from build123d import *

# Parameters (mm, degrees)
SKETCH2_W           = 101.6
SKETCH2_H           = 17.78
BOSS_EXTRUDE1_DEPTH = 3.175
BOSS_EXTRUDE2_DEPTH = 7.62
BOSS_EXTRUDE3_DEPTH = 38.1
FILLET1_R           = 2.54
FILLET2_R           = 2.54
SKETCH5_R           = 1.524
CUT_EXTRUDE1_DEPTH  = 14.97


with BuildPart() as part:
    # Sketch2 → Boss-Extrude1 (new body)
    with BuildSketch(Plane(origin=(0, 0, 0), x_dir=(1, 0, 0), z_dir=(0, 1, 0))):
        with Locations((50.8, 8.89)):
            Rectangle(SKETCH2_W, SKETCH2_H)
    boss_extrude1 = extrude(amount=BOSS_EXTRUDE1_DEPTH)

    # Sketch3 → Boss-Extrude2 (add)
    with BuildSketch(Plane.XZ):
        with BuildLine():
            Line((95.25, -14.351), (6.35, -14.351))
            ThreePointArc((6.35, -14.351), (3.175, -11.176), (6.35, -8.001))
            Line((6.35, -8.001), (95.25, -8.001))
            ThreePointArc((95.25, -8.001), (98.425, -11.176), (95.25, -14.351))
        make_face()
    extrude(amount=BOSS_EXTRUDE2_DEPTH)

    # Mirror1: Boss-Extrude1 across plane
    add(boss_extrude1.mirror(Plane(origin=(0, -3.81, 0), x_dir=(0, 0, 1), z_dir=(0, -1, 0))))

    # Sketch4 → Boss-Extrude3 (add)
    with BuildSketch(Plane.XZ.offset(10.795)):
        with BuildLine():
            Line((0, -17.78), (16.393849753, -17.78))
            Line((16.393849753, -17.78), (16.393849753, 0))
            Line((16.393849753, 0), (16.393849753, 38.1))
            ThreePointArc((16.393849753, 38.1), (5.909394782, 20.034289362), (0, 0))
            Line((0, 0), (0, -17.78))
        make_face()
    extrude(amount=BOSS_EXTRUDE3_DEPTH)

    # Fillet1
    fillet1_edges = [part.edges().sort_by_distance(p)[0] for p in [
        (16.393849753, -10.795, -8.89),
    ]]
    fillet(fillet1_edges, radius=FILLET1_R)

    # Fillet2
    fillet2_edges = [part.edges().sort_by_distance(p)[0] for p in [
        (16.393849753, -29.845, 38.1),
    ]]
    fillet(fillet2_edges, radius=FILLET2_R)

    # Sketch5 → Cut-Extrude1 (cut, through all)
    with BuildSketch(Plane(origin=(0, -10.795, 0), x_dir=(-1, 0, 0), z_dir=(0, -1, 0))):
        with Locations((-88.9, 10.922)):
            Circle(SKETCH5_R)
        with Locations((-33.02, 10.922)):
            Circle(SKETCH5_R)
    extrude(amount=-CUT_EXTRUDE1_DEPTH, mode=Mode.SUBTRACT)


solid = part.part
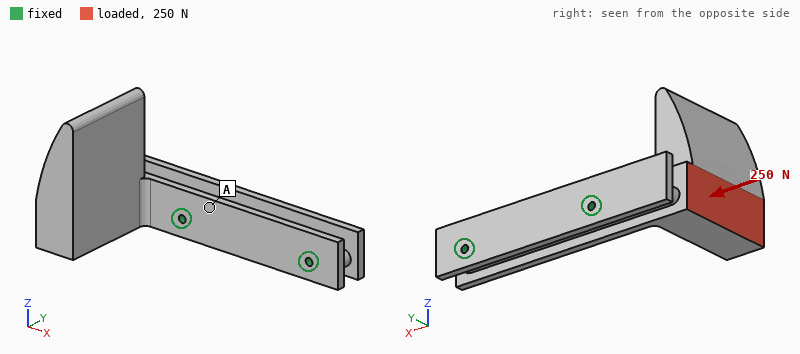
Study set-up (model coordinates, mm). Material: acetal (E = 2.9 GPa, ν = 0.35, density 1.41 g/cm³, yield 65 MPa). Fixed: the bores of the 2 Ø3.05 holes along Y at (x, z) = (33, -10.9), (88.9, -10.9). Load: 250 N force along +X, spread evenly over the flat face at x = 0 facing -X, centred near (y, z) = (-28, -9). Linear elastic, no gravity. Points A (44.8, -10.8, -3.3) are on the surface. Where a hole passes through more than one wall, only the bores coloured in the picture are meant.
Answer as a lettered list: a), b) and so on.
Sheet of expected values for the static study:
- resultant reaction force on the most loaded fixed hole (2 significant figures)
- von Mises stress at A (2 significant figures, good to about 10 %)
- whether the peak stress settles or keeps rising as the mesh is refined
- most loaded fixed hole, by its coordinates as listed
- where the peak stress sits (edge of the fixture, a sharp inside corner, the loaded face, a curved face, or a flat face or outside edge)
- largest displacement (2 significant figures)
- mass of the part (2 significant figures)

a) 230 N
b) 2.4 MPa
c) keeps rising
d) (33, -10.9)
e) edge of the fixture
f) 1.1 mm
g) 58 g
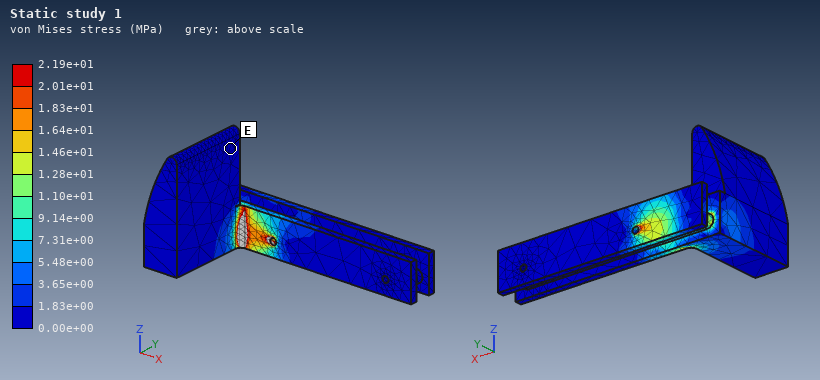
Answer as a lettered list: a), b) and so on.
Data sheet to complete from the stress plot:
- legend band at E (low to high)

a) 0.00e+00 to 1.83e+00 MPa
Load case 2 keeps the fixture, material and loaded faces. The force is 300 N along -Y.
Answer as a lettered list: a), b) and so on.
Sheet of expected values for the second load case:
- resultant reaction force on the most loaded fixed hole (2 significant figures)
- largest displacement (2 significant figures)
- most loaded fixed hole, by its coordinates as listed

a) 330 N
b) 1.4 mm
c) (33, -10.9)
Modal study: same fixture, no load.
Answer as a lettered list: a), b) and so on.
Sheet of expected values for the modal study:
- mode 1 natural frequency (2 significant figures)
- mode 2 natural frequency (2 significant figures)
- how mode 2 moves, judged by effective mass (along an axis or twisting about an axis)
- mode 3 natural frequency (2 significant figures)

a) 220 Hz
b) 410 Hz
c) along X
d) 800 Hz
